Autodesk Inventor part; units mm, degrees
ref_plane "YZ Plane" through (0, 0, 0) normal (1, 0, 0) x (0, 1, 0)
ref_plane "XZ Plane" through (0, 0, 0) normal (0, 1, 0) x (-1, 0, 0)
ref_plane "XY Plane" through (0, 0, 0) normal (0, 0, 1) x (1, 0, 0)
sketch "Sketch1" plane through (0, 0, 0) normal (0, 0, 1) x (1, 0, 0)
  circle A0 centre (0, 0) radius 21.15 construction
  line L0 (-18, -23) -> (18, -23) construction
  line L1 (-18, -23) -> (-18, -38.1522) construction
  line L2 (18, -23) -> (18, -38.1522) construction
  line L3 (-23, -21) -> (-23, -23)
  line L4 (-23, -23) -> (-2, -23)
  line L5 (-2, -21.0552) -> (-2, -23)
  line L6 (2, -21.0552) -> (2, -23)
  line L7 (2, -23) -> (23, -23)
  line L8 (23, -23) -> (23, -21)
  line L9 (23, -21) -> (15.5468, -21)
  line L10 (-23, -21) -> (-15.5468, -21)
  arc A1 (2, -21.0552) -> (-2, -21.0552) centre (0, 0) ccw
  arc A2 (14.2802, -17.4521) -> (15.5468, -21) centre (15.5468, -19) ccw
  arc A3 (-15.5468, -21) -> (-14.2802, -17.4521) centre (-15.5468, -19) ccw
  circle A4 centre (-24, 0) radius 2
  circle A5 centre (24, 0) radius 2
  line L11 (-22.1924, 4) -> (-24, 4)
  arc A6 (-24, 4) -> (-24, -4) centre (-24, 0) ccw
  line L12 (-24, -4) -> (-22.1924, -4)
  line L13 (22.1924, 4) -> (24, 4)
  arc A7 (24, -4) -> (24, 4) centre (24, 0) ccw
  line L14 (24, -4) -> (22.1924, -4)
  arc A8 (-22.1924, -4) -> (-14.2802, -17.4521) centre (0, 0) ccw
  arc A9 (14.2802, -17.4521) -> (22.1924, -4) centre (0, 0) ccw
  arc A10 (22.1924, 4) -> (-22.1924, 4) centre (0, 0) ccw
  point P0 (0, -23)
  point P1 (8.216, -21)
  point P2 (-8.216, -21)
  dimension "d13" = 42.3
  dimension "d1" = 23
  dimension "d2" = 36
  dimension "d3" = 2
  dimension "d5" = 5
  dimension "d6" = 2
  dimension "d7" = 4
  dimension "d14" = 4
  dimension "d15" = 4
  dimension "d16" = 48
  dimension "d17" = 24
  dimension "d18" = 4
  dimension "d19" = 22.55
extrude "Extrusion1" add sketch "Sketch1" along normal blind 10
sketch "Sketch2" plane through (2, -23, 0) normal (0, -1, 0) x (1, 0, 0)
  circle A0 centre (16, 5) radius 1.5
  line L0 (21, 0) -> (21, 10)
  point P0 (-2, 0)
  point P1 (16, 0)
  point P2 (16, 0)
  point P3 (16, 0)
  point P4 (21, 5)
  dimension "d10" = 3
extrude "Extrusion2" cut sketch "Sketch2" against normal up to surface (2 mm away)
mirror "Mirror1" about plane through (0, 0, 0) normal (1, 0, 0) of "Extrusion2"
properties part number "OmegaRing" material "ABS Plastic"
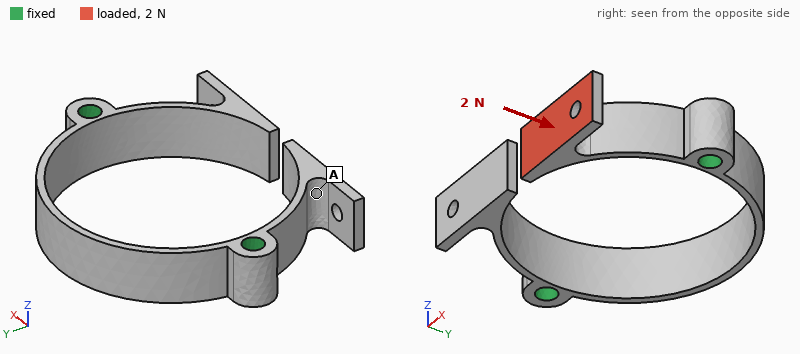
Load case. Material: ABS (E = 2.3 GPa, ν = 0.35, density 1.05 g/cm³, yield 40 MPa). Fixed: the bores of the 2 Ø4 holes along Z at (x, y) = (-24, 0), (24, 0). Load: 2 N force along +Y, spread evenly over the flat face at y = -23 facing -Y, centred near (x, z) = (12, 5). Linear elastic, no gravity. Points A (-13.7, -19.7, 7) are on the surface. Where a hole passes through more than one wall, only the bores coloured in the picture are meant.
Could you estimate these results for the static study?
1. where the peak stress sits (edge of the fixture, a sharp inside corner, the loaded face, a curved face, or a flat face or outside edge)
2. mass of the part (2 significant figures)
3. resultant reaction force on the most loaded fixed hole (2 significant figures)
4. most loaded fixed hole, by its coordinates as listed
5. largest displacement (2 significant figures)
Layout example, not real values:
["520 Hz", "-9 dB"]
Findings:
["a curved face", "3.4 g", "2.0 N", "(24, 0)", "0.83 mm"]
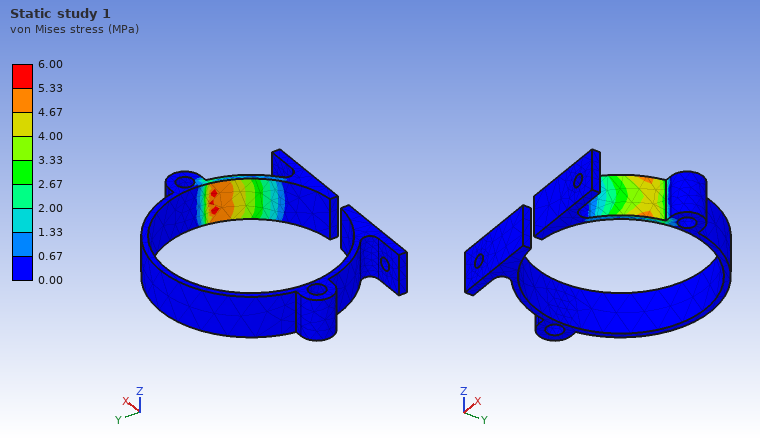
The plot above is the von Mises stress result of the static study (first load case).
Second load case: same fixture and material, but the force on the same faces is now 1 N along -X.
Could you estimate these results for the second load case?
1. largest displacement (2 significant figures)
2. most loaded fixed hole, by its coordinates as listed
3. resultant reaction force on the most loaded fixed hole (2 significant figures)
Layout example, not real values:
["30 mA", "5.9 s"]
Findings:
["0.83 mm", "(24, 0)", "1.0 N"]
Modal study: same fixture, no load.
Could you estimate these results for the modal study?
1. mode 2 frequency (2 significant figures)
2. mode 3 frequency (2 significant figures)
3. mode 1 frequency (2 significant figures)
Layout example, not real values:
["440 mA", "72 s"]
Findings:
["250 Hz", "810 Hz", "250 Hz"]
